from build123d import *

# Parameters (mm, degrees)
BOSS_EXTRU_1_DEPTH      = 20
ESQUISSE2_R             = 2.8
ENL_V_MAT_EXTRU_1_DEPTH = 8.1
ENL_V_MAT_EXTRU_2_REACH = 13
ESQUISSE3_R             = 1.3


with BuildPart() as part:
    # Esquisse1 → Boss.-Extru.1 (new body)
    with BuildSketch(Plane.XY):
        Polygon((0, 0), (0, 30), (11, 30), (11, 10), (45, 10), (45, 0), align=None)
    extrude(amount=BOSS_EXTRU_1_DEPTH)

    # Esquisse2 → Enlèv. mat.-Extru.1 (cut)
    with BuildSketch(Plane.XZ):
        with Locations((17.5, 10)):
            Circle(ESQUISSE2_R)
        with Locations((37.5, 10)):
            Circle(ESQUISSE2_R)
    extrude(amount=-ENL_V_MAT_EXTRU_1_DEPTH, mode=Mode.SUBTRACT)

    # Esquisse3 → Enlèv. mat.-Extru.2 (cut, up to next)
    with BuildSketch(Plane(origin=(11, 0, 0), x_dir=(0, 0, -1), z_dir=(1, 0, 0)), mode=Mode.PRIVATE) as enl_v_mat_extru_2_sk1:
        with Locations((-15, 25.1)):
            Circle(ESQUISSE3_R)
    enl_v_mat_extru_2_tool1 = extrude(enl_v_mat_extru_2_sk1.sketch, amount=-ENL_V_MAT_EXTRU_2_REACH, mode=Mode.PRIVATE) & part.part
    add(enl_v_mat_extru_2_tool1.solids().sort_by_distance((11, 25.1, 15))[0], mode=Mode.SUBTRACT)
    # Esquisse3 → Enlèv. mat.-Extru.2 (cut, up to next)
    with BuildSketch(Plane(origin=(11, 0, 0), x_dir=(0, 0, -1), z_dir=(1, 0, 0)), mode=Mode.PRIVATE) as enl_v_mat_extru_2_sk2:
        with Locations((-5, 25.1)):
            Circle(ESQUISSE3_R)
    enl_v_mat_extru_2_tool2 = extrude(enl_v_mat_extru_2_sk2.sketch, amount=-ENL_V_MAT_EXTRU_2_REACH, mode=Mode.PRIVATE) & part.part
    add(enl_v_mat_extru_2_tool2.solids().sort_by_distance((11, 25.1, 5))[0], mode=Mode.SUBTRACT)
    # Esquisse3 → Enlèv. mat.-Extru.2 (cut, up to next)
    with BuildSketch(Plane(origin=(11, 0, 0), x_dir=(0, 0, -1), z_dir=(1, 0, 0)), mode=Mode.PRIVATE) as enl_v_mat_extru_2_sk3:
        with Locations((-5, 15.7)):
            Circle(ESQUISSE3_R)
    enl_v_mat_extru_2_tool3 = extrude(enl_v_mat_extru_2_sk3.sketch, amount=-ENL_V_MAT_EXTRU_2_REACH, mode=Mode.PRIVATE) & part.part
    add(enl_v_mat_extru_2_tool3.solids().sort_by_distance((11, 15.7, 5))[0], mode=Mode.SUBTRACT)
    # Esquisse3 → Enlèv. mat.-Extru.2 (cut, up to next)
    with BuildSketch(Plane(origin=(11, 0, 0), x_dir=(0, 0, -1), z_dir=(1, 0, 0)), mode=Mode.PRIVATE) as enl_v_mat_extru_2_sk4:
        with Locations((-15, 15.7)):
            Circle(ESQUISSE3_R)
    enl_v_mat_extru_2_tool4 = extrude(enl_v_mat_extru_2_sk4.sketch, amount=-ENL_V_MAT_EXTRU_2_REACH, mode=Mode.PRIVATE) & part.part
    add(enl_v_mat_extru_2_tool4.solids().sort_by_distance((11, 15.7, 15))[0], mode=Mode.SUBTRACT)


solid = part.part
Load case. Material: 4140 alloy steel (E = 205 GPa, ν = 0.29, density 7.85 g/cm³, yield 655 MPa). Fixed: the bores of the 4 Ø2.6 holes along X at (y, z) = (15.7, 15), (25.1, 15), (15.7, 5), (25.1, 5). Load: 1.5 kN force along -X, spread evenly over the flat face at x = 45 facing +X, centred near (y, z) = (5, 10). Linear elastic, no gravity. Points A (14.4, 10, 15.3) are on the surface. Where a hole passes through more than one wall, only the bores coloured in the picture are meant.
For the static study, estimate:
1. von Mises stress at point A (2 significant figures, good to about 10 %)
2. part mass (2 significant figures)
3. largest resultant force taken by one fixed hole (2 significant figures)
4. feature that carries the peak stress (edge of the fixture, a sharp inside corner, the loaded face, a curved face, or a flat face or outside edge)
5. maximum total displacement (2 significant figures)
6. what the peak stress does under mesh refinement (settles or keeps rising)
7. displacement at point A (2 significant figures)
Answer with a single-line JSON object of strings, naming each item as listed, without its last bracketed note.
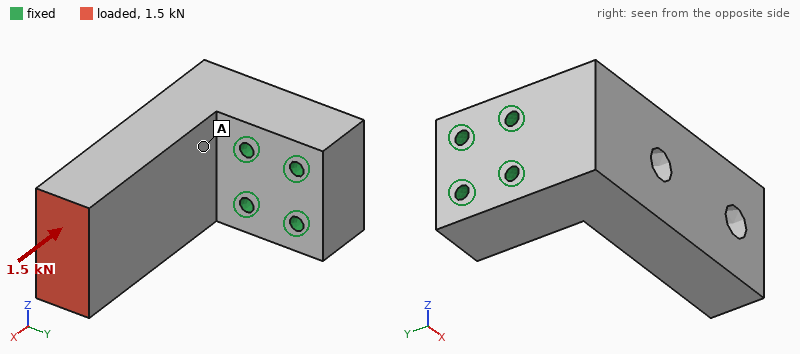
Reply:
{"von Mises stress at point A": "9.7 MPa", "part mass": "100 g", "largest resultant force taken by one fixed hole": "830 N", "feature that carries the peak stress": "edge of the fixture", "maximum total displacement": "12 µm", "what the peak stress does under mesh refinement": "keeps rising", "displacement at point A": "2.4 µm"}
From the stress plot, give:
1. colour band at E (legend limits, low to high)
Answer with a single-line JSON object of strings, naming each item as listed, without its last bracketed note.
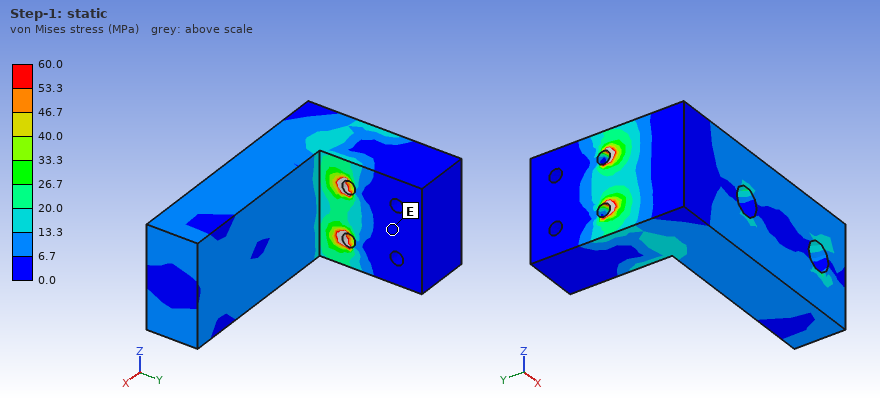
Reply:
{"colour band at E": "0.0 to 6.7 MPa"}
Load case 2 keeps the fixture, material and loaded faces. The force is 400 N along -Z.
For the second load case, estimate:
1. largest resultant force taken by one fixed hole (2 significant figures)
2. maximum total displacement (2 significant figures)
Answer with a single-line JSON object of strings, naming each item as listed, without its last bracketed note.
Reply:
{"largest resultant force taken by one fixed hole": "910 N", "maximum total displacement": "16 µm"}
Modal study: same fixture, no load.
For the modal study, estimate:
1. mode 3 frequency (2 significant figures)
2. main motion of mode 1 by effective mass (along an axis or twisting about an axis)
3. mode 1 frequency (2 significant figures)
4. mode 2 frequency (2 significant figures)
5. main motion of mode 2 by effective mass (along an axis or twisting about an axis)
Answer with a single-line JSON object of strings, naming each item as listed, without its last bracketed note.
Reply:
{"mode 3 frequency": "15 kHz", "main motion of mode 1 by effective mass": "along Y", "mode 1 frequency": "4100 Hz", "mode 2 frequency": "6000 Hz", "main motion of mode 2 by effective mass": "along Z"}
